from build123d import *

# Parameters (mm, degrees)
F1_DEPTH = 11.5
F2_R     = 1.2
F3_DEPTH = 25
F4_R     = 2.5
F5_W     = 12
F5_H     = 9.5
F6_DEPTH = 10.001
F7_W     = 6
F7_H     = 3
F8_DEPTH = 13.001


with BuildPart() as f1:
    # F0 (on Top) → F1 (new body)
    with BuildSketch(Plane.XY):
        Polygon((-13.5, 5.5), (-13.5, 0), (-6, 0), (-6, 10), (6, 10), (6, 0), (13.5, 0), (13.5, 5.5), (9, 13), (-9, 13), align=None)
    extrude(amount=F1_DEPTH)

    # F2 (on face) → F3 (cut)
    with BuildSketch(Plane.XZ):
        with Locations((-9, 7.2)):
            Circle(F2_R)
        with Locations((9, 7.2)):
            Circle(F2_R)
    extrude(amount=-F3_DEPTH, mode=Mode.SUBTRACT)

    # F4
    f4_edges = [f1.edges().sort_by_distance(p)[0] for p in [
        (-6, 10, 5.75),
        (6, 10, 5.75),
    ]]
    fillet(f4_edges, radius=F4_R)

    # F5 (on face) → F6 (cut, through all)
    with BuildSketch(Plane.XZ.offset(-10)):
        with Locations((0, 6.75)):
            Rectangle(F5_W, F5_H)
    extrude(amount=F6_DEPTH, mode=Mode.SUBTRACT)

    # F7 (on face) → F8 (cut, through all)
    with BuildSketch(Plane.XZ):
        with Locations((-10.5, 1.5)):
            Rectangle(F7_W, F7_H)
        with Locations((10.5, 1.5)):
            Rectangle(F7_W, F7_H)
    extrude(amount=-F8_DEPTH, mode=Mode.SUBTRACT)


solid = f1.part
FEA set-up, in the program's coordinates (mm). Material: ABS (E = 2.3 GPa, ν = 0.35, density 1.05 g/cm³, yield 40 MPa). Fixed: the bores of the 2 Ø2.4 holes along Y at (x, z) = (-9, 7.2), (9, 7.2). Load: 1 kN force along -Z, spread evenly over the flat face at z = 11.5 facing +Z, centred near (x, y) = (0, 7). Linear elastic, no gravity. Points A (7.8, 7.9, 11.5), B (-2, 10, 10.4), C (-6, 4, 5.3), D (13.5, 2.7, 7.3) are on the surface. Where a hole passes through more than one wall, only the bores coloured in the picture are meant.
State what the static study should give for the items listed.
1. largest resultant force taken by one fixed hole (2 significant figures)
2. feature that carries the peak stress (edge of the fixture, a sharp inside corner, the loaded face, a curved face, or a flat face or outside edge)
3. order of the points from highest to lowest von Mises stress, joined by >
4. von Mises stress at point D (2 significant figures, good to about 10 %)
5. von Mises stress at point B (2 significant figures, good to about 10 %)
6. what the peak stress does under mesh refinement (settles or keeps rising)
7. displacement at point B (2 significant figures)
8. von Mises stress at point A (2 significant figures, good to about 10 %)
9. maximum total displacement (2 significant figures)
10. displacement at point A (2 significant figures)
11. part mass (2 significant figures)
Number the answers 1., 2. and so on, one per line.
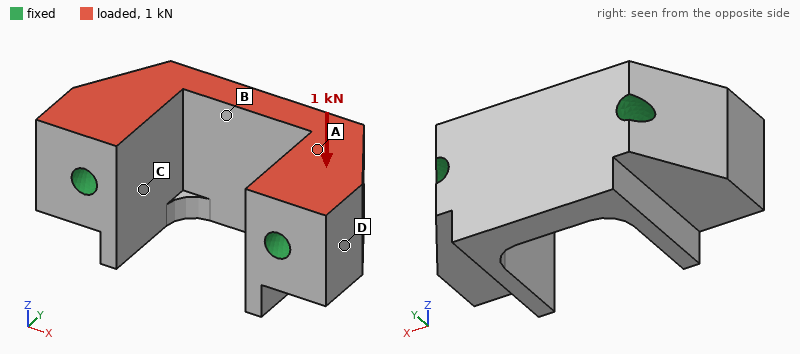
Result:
1. 500 N
2. edge of the fixture
3. A > B > D > C
4. 2.8 MPa
5. 5.2 MPa
6. keeps rising
7. 34 µm
8. 7.2 MPa
9. 40 µm
10. 11 µm
11. 1.9 g
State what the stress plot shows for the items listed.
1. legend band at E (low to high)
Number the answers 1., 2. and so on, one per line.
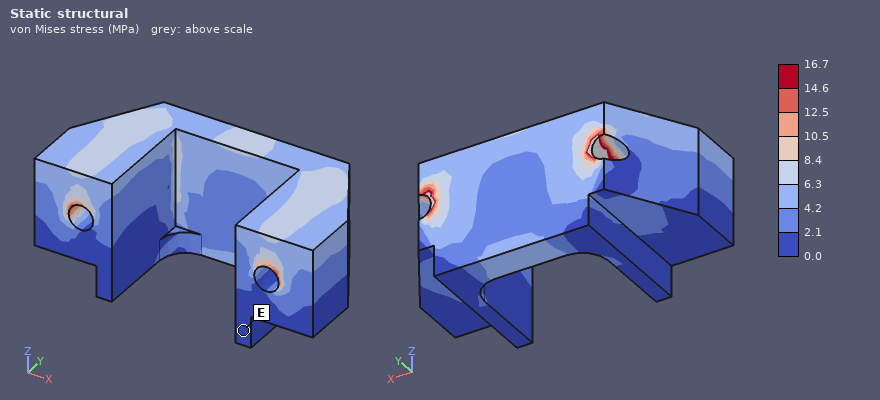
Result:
1. 0.0 to 2.1 MPa
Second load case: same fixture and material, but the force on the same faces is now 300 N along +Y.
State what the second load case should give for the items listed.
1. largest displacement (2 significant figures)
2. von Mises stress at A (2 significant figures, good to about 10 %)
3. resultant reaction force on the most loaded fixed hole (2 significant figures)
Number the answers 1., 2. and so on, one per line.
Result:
1. 61 µm
2. 3.5 MPa
3. 150 N
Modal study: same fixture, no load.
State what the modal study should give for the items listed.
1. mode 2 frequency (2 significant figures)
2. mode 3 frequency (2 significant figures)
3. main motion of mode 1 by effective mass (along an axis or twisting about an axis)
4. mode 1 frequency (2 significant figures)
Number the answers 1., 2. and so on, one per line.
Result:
1. 19 kHz
2. 20 kHz
3. along Y
4. 15 kHz
